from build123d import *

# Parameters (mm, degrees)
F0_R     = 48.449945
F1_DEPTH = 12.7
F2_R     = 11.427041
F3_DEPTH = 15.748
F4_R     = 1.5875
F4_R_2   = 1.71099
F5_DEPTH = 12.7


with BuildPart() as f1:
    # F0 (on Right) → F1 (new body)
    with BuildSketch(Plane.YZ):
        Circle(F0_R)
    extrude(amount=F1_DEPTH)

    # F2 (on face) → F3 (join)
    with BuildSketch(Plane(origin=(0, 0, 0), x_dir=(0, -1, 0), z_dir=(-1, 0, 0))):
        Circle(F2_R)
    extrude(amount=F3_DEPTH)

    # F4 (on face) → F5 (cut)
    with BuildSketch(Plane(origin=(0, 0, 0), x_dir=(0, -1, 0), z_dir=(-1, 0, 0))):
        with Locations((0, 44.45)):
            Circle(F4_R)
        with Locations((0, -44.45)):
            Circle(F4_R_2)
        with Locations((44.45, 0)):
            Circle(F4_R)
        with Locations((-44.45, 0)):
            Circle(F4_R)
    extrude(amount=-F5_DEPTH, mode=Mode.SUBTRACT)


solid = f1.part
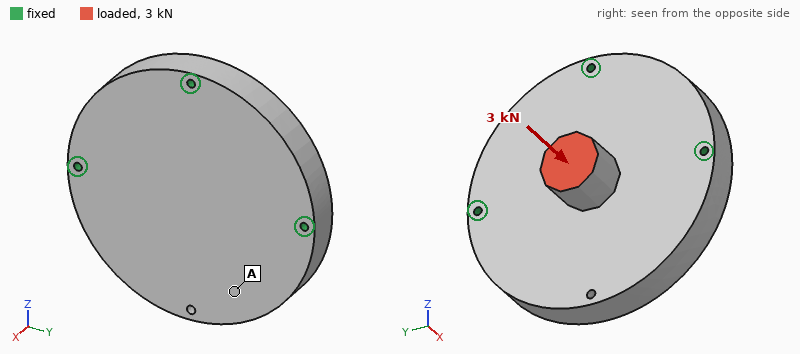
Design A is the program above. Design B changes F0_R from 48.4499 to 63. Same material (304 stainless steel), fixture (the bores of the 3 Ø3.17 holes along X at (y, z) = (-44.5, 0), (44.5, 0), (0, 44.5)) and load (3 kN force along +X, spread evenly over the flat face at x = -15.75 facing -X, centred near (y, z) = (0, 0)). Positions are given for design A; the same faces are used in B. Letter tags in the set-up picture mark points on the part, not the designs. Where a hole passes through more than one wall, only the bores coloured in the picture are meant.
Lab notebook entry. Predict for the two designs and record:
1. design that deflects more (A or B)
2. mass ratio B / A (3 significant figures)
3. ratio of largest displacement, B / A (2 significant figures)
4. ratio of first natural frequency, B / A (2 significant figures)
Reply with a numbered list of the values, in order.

1. A
2. 1.65
3. 0.86
4. 0.72
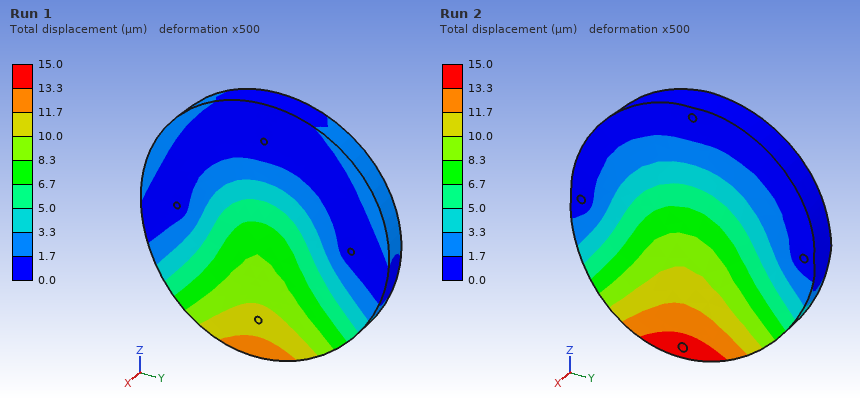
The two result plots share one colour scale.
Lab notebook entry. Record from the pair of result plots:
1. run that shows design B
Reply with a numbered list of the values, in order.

1. Run 1
